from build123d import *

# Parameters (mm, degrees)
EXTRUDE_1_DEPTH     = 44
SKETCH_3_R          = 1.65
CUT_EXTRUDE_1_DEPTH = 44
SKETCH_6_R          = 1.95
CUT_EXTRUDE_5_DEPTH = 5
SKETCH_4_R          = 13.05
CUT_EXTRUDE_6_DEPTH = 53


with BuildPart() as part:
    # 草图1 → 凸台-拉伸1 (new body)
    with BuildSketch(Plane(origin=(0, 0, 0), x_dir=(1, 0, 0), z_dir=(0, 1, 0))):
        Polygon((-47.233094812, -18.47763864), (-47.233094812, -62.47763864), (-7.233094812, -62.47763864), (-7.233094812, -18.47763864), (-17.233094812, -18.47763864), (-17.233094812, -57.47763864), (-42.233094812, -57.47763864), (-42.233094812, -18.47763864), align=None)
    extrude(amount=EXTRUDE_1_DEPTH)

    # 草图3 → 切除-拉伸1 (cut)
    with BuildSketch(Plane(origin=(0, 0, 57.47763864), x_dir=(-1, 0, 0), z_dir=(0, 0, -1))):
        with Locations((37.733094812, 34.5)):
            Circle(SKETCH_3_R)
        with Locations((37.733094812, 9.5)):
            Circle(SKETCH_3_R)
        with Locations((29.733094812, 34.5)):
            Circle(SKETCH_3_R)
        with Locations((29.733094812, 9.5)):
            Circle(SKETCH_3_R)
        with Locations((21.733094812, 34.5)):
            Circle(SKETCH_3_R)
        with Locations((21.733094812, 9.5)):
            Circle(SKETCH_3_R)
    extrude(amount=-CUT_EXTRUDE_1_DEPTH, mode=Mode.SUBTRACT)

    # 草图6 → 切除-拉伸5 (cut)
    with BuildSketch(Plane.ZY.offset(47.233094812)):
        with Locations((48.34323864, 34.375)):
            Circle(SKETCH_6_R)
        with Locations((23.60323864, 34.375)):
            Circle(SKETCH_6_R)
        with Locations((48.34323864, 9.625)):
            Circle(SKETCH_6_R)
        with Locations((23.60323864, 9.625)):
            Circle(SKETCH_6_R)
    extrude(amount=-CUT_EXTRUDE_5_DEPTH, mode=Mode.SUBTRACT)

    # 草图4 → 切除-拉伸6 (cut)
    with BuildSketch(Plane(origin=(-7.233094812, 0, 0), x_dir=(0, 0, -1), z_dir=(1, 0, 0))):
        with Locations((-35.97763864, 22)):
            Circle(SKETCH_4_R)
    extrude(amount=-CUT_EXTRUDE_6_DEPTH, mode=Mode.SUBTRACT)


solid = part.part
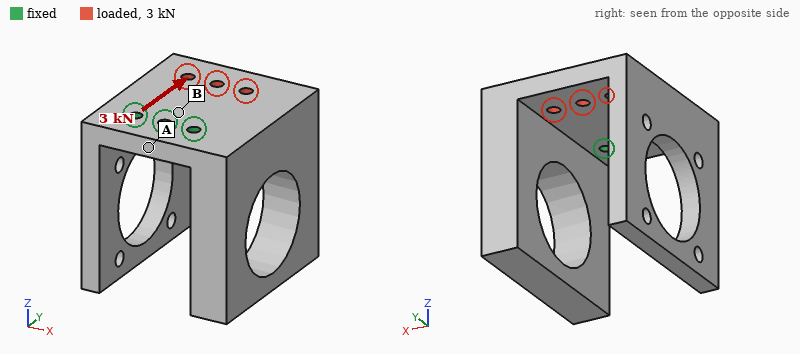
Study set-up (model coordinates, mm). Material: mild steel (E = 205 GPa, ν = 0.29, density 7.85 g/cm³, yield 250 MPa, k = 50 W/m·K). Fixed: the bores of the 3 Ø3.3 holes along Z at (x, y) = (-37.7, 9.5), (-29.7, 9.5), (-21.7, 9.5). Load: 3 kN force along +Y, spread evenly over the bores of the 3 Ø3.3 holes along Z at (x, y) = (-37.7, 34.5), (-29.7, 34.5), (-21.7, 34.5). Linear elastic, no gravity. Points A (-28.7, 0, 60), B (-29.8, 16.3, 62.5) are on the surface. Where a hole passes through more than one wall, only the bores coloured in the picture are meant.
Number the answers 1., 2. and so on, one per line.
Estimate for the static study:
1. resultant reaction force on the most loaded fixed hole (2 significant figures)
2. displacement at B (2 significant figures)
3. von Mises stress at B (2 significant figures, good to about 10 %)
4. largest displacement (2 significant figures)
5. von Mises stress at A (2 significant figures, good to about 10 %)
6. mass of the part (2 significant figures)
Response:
1. 1.2 kN
2. 0.63 µm
3. 23 MPa
4. 3.2 µm
5. 6.8 MPa
6. 200 g
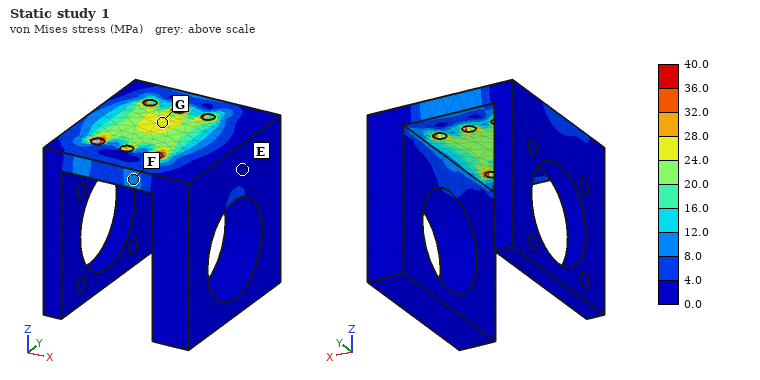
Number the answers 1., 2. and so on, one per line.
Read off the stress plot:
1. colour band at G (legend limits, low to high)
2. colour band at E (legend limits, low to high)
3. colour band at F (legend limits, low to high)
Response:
1. 24.0 to 28.0 MPa
2. 0.0 to 4.0 MPa
3. 8.0 to 12.0 MPa
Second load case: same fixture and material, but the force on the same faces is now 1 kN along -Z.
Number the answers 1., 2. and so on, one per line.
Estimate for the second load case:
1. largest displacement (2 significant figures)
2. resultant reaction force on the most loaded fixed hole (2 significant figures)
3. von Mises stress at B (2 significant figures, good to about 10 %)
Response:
1. 63 µm
2. 380 N
3. 59 MPa
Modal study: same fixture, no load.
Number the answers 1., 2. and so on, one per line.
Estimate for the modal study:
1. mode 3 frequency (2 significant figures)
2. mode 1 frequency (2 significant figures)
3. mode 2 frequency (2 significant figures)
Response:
1. 1900 Hz
2. 1500 Hz
3. 1800 Hz
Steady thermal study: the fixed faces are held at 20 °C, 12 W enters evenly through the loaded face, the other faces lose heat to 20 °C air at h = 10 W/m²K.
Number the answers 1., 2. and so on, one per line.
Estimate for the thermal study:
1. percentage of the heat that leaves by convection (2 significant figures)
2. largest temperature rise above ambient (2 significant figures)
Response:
1. 11 %
2. 28 K
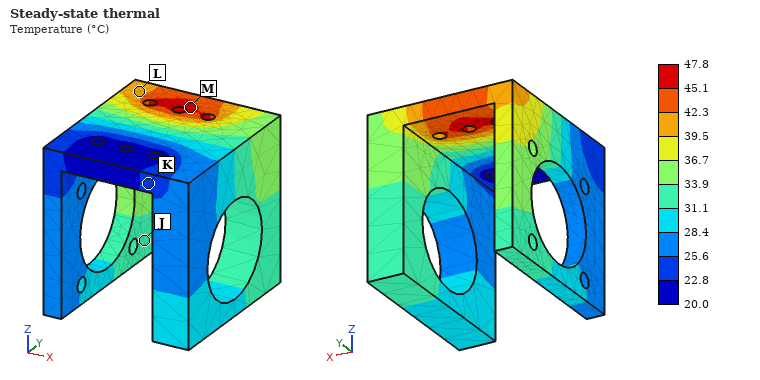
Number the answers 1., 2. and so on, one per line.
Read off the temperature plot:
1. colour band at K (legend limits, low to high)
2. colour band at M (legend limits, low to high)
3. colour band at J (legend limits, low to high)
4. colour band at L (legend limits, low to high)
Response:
1. 22.8 to 25.6 °C
2. 45.1 to 47.8 °C
3. 31.1 to 33.9 °C
4. 39.5 to 42.3 °C
